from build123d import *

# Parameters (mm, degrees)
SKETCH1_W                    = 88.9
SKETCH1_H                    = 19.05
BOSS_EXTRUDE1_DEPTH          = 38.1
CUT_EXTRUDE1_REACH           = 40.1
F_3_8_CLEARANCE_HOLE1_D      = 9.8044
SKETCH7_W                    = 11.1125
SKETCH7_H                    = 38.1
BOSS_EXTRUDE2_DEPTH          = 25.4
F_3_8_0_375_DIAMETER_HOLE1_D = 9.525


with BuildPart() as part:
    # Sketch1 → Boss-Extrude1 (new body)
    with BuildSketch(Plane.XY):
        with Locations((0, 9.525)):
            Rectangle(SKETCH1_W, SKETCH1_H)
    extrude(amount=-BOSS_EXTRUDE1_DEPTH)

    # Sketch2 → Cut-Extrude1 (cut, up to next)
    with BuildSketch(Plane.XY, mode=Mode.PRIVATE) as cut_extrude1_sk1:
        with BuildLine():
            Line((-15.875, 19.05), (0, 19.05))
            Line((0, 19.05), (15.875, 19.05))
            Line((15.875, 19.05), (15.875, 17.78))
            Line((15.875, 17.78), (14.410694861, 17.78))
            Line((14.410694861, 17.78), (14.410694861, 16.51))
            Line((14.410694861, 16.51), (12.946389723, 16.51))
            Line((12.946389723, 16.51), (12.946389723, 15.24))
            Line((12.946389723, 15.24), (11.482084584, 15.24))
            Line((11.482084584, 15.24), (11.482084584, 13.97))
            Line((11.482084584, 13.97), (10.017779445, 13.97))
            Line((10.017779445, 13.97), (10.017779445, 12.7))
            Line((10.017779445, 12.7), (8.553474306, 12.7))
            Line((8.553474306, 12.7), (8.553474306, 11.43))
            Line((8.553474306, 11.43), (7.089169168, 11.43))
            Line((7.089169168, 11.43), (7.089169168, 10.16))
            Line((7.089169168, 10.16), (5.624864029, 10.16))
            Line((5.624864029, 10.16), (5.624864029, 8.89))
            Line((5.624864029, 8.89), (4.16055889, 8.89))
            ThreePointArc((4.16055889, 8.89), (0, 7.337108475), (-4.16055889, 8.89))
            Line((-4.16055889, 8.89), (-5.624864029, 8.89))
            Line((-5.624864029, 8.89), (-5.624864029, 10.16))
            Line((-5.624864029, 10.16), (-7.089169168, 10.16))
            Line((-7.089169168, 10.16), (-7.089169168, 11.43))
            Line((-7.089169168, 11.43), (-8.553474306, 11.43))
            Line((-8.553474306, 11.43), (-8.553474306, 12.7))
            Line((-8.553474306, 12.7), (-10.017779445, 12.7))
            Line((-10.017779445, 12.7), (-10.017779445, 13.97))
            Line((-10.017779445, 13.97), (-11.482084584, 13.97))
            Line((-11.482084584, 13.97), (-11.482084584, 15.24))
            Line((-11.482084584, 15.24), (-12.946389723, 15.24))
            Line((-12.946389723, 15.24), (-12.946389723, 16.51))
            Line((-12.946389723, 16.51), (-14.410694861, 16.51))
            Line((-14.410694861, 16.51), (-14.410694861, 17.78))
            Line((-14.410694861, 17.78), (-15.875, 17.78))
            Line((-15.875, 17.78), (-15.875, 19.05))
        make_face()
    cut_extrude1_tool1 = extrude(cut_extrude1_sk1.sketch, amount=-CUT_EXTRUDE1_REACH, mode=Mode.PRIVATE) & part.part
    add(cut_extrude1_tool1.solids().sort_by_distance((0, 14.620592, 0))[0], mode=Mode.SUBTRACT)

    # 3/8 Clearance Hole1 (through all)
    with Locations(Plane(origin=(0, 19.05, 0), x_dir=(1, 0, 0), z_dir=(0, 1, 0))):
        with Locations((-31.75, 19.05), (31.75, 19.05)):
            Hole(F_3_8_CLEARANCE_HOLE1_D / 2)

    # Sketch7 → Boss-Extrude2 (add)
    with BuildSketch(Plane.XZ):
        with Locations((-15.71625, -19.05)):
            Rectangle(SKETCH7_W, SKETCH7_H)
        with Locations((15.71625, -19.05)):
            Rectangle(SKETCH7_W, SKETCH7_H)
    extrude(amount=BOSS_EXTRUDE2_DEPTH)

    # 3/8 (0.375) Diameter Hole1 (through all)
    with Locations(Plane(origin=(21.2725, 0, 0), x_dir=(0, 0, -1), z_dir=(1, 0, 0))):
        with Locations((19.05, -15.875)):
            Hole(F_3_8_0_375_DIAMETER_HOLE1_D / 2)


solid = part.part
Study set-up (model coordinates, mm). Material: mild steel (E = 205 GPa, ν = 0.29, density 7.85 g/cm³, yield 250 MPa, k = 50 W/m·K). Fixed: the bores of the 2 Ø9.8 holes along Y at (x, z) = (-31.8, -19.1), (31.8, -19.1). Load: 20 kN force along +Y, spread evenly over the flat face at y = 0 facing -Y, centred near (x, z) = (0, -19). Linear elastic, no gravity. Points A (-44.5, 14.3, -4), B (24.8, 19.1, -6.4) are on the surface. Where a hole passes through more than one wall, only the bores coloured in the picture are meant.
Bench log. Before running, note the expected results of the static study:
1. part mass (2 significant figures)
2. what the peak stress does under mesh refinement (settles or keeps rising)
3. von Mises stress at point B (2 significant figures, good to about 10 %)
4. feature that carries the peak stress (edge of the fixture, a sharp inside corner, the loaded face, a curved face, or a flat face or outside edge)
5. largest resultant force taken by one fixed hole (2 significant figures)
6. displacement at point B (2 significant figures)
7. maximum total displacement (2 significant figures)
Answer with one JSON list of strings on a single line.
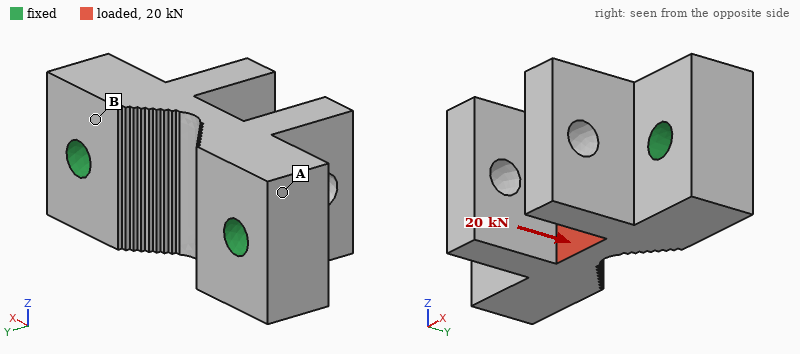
["570 g", "keeps rising", "37 MPa", "edge of the fixture", "13 kN", "5.4 µm", "23 µm"]
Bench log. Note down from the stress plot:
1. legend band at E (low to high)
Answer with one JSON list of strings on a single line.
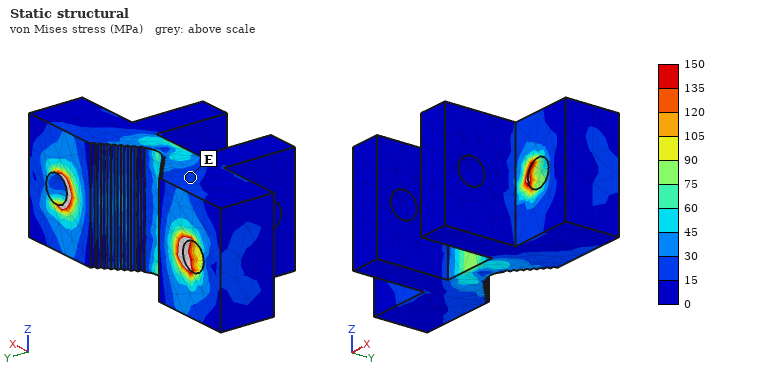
["15 to 30 MPa"]
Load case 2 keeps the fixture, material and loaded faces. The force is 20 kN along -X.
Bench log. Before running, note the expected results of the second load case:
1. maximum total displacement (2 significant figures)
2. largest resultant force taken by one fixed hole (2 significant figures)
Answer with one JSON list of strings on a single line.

["4.2 µm", "11 kN"]
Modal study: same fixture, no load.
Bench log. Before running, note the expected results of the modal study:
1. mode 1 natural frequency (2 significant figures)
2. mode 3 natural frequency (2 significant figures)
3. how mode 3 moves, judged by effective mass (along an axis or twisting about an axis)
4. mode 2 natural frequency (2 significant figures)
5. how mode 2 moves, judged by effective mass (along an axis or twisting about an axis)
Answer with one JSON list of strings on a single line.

["8500 Hz", "9800 Hz", "along X", "9300 Hz", "along Z"]
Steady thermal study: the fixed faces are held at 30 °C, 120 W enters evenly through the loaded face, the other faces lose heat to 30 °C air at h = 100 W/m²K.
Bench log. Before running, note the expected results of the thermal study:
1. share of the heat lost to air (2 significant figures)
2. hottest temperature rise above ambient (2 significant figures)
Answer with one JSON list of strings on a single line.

["22 %", "58 K"]
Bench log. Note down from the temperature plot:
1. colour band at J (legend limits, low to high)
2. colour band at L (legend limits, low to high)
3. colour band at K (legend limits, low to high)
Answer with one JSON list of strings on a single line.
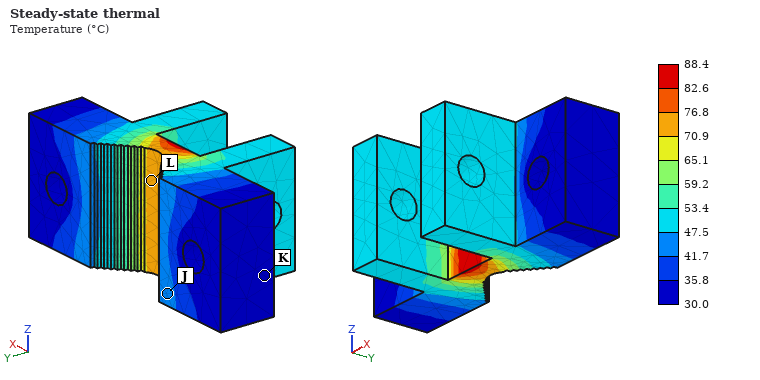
["41.7 to 47.5 °C", "70.9 to 76.8 °C", "30.0 to 35.8 °C"]
